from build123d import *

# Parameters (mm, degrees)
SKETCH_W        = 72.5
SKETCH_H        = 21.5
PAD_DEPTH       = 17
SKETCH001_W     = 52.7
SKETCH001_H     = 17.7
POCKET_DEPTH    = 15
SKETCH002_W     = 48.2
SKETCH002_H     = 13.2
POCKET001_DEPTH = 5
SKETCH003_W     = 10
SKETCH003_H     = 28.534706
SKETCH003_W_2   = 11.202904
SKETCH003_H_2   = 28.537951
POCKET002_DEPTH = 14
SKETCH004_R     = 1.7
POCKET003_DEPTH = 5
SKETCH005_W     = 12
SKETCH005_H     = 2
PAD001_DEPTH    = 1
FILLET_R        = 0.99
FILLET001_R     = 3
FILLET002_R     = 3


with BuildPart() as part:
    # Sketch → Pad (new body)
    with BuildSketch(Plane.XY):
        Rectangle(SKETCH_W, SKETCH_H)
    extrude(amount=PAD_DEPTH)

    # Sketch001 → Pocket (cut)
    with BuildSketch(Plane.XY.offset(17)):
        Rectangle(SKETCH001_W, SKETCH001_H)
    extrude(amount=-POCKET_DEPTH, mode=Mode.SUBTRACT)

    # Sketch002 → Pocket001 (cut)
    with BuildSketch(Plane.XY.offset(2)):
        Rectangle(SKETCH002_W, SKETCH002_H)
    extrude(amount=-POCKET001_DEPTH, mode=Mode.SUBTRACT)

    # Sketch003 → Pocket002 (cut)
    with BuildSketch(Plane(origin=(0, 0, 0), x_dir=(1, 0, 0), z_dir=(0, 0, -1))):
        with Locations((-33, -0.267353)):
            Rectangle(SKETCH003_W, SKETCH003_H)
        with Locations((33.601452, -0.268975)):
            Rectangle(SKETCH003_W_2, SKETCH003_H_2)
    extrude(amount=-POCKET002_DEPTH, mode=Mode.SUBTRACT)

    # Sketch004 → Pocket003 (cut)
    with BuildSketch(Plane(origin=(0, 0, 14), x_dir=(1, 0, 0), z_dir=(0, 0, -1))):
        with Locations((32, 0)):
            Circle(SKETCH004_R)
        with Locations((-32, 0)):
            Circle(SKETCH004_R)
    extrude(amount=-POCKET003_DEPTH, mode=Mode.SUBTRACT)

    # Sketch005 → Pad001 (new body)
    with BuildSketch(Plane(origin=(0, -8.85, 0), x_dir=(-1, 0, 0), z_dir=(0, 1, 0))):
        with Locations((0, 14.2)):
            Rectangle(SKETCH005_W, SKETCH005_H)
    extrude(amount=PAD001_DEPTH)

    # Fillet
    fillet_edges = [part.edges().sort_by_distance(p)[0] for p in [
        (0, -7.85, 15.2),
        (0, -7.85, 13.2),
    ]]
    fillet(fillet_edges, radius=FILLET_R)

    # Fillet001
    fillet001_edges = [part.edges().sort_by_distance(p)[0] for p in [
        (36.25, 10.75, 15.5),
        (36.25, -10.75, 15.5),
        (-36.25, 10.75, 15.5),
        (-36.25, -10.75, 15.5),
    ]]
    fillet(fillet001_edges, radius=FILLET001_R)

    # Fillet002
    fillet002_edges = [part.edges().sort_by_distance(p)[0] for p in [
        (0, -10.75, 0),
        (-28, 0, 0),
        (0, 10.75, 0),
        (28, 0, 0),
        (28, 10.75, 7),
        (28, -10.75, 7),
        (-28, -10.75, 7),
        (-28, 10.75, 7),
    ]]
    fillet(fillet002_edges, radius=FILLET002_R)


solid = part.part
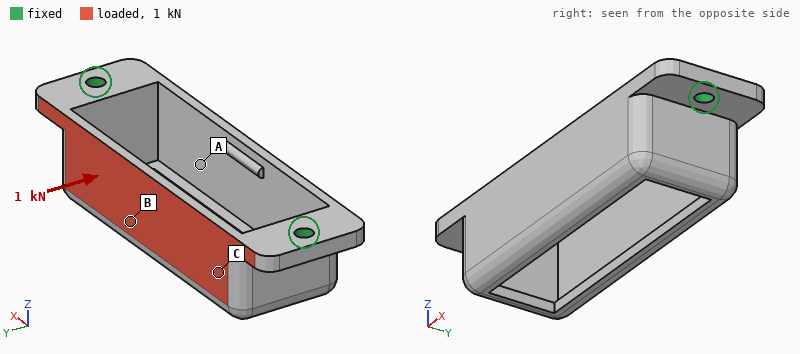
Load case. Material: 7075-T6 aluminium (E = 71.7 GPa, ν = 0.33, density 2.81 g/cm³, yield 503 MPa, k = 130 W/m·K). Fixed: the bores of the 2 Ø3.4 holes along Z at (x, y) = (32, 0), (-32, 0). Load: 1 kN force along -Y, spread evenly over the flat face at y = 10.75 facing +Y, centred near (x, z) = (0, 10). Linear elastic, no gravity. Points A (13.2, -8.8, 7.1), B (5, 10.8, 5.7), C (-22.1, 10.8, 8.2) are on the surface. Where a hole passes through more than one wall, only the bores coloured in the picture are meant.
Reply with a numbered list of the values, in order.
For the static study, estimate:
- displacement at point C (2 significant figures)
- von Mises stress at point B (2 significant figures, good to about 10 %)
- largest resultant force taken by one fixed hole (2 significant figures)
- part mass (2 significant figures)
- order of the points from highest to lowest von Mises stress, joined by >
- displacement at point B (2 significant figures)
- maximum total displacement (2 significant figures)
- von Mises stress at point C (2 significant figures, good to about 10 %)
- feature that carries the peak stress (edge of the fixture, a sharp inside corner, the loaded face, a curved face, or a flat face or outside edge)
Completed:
1. 0.12 mm
2. 170 MPa
3. 610 N
4. 16 g
5. B > C > A
6. 0.43 mm
7. 0.66 mm
8. 110 MPa
9. the loaded face
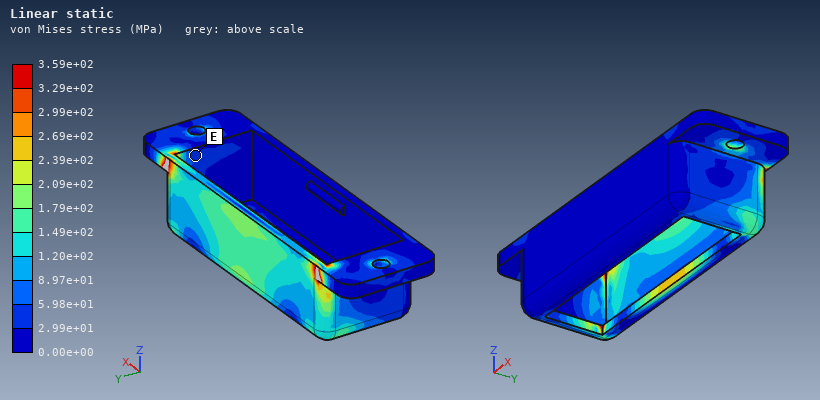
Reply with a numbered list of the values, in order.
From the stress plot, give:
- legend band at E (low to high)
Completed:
1. 2.99e+01 to 5.98e+01 MPa
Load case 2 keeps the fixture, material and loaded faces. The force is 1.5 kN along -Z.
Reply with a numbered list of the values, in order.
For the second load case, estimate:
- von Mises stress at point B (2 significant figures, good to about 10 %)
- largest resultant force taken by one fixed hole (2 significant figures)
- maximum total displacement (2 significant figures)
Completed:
1. 52 MPa
2. 880 N
3. 0.19 mm
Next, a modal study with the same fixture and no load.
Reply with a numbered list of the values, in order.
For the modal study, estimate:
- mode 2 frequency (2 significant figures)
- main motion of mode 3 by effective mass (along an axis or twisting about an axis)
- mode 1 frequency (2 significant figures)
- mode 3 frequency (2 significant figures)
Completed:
1. 3600 Hz
2. twisting about X
3. 3500 Hz
4. 5100 Hz
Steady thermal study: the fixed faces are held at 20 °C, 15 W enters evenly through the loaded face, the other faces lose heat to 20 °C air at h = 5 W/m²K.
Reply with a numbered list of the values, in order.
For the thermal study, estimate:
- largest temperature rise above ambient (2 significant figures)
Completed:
1. 42 K
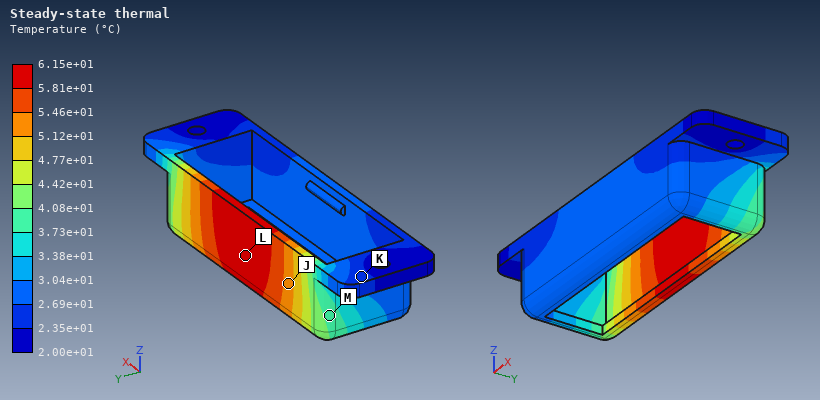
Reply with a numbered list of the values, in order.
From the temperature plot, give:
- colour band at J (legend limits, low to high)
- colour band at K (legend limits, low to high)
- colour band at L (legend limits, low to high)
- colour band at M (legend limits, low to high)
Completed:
1. 5.12e+01 to 5.46e+01 °C
2. 2.35e+01 to 2.69e+01 °C
3. 5.81e+01 to 6.15e+01 °C
4. 3.73e+01 to 4.08e+01 °C
